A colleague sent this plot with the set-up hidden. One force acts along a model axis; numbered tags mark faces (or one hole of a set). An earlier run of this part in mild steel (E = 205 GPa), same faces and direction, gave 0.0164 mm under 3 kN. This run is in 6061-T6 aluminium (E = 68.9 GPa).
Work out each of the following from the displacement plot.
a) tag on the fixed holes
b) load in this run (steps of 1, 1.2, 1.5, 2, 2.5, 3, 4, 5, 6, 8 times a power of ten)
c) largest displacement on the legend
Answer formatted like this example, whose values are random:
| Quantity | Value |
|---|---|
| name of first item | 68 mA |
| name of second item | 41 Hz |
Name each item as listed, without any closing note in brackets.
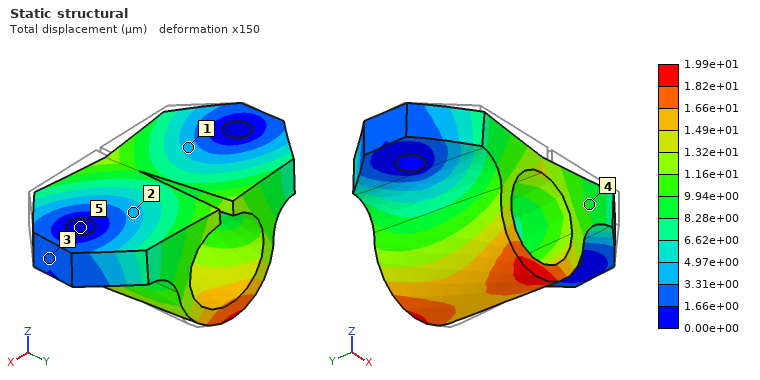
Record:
| Quantity | Value |
|---|---|
| tag on the fixed holes | 5 |
| load in this run | 1.2 kN |
| largest displacement on the legend | 1.99e+01 µm |
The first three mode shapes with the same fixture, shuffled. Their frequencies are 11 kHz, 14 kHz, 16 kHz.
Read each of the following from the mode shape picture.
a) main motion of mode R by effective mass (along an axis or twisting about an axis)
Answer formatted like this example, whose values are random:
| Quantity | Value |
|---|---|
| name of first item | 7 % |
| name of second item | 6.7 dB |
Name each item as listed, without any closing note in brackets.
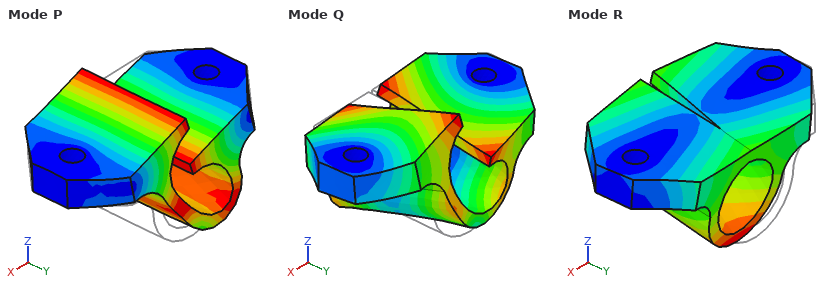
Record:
| Quantity | Value |
|---|---|
| main motion of mode R by effective mass | along Y |
